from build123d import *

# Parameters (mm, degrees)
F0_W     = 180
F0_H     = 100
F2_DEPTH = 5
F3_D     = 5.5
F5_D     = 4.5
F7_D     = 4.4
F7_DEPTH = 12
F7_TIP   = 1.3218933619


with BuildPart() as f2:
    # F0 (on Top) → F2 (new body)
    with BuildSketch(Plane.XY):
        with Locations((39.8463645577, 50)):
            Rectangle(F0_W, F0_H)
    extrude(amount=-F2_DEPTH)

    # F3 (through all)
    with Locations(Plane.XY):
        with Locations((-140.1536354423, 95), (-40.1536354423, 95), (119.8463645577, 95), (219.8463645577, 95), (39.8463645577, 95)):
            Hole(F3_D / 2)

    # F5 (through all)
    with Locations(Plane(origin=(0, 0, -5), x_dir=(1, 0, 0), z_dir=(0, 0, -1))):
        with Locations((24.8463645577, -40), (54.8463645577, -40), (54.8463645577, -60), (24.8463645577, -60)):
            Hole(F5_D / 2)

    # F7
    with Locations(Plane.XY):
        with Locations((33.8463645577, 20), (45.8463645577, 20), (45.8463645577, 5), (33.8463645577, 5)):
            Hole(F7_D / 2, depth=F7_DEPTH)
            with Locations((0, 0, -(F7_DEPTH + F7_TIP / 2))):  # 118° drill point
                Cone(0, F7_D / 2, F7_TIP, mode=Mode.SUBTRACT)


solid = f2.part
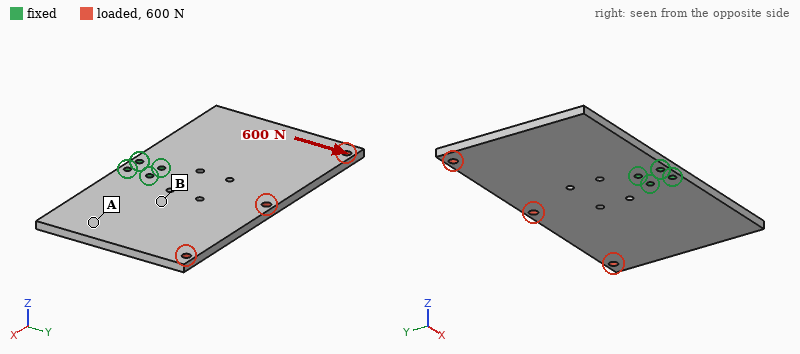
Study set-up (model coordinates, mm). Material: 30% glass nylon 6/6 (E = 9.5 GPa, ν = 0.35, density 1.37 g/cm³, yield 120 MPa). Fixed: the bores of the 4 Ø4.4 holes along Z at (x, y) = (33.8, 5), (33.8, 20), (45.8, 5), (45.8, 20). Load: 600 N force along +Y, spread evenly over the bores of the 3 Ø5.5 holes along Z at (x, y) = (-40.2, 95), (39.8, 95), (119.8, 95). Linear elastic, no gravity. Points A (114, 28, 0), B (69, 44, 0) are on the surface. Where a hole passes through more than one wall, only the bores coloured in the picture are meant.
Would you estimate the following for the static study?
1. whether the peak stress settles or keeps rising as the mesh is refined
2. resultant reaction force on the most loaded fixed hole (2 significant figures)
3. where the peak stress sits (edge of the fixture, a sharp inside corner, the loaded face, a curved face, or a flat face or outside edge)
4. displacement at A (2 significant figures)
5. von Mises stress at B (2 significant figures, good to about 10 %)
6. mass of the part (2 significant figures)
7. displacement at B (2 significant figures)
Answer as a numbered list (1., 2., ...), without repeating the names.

1. keeps rising
2. 220 N
3. edge of the fixture
4. 21 µm
5. 1.3 MPa
6. 120 g
7. 10 µm
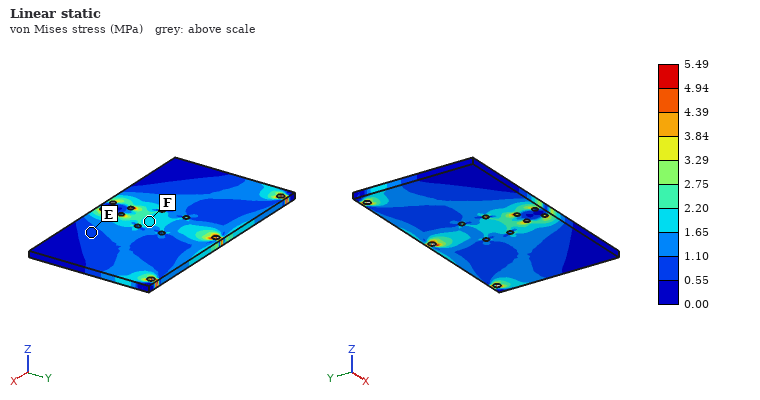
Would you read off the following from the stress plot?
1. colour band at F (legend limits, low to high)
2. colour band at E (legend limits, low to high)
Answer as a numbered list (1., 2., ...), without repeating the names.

1. 1.65 to 2.20 MPa
2. 0.55 to 1.10 MPa
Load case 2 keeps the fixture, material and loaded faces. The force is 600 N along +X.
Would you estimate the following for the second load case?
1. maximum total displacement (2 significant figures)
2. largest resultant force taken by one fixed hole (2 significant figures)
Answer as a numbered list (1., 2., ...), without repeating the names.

1. 0.38 mm
2. 1.4 kN
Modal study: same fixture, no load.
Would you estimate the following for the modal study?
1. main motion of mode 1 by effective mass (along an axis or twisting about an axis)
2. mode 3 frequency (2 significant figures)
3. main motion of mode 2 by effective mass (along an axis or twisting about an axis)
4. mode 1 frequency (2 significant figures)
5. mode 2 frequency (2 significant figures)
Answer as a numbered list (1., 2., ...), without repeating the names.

1. twisting about Y
2. 350 Hz
3. along Z
4. 190 Hz
5. 220 Hz
